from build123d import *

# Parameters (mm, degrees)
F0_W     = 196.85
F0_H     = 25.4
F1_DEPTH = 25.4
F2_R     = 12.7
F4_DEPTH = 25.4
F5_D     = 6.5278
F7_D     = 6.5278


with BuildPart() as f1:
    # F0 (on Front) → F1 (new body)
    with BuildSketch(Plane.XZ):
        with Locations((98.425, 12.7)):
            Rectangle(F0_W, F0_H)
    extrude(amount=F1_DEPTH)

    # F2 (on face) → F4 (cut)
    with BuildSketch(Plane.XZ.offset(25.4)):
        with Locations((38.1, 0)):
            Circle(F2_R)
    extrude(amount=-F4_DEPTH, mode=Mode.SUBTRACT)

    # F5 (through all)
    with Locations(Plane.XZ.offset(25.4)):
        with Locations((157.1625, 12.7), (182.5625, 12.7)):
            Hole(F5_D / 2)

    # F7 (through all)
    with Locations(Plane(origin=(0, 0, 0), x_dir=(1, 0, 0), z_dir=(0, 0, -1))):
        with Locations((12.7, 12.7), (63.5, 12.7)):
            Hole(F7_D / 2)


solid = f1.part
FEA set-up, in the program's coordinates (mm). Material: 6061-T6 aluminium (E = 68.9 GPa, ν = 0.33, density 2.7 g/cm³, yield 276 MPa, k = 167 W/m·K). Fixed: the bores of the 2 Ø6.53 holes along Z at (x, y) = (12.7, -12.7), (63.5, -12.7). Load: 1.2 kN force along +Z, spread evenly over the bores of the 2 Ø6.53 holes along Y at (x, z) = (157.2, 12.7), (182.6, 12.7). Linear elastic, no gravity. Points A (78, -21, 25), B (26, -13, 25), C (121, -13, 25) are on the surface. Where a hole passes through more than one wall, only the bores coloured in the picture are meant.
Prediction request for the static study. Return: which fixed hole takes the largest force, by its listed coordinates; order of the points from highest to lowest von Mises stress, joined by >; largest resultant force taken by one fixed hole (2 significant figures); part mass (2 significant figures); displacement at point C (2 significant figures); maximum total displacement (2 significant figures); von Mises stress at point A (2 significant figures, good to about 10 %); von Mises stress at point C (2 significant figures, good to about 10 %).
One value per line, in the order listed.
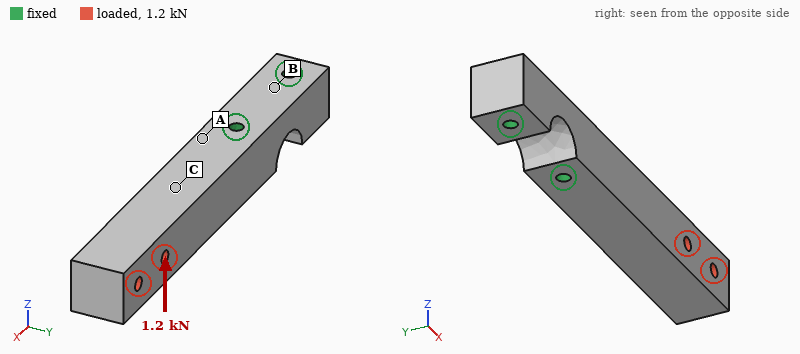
(63.5, -12.7)
A > C > B
1.6 kN
320 g
0.089 mm
0.30 mm
39 MPa
21 MPa
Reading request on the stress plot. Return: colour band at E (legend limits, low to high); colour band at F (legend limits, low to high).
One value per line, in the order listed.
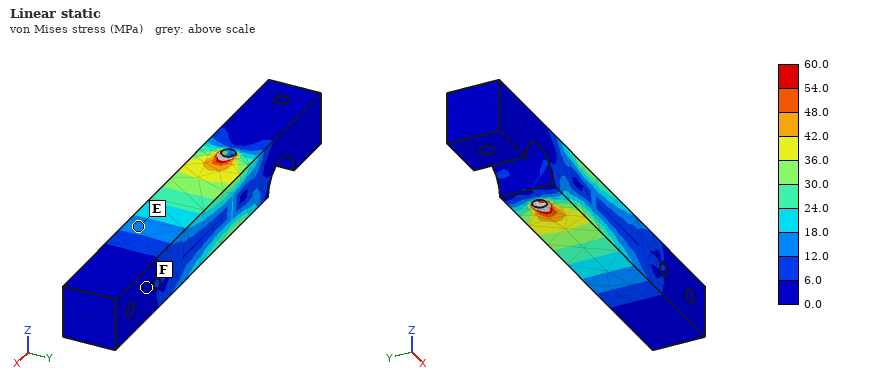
12.0 to 18.0 MPa
0.0 to 6.0 MPa
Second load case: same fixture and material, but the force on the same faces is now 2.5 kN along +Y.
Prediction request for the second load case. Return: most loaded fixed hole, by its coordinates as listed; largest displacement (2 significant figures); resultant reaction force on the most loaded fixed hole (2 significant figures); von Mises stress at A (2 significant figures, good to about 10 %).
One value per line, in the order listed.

(63.5, -12.7)
0.80 mm
5.2 kN
57 MPa
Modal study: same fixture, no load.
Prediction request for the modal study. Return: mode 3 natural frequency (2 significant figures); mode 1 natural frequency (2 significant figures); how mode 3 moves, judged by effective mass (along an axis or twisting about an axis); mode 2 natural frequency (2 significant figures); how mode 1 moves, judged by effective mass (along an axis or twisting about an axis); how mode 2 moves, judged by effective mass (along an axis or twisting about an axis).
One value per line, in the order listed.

5300 Hz
990 Hz
twisting about X
1100 Hz
along Y
along Z
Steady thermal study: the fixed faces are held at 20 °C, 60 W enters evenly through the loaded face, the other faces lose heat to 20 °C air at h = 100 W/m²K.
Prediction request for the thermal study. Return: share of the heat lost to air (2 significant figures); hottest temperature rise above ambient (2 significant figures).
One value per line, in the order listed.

49 %
37 K
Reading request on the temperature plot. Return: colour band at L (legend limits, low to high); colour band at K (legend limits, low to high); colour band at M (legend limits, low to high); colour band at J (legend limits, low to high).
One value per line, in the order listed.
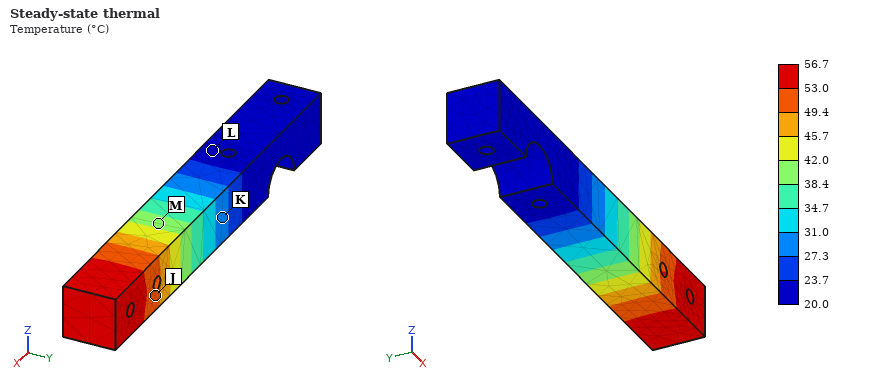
20.0 to 23.7 °C
27.3 to 31.0 °C
38.4 to 42.0 °C
49.4 to 53.0 °C
